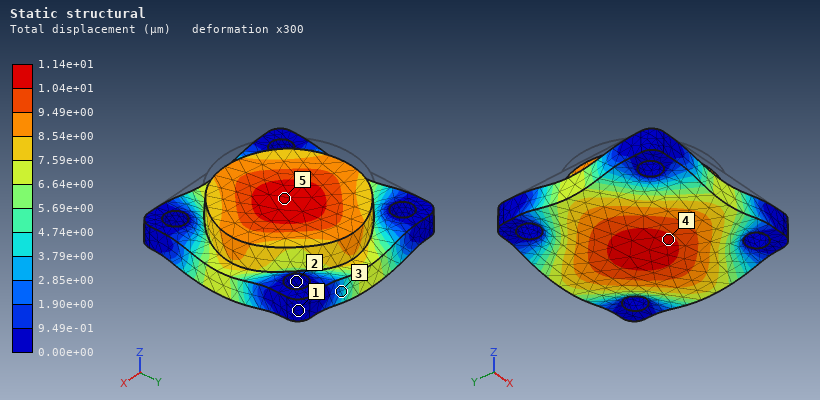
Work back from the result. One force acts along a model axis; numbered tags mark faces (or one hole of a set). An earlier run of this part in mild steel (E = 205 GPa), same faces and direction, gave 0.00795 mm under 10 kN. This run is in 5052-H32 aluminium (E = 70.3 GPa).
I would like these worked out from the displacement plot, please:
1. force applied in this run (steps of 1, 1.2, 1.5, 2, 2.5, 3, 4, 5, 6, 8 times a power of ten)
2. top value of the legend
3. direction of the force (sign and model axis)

5 kN
1.14e+01 µm
-Z
